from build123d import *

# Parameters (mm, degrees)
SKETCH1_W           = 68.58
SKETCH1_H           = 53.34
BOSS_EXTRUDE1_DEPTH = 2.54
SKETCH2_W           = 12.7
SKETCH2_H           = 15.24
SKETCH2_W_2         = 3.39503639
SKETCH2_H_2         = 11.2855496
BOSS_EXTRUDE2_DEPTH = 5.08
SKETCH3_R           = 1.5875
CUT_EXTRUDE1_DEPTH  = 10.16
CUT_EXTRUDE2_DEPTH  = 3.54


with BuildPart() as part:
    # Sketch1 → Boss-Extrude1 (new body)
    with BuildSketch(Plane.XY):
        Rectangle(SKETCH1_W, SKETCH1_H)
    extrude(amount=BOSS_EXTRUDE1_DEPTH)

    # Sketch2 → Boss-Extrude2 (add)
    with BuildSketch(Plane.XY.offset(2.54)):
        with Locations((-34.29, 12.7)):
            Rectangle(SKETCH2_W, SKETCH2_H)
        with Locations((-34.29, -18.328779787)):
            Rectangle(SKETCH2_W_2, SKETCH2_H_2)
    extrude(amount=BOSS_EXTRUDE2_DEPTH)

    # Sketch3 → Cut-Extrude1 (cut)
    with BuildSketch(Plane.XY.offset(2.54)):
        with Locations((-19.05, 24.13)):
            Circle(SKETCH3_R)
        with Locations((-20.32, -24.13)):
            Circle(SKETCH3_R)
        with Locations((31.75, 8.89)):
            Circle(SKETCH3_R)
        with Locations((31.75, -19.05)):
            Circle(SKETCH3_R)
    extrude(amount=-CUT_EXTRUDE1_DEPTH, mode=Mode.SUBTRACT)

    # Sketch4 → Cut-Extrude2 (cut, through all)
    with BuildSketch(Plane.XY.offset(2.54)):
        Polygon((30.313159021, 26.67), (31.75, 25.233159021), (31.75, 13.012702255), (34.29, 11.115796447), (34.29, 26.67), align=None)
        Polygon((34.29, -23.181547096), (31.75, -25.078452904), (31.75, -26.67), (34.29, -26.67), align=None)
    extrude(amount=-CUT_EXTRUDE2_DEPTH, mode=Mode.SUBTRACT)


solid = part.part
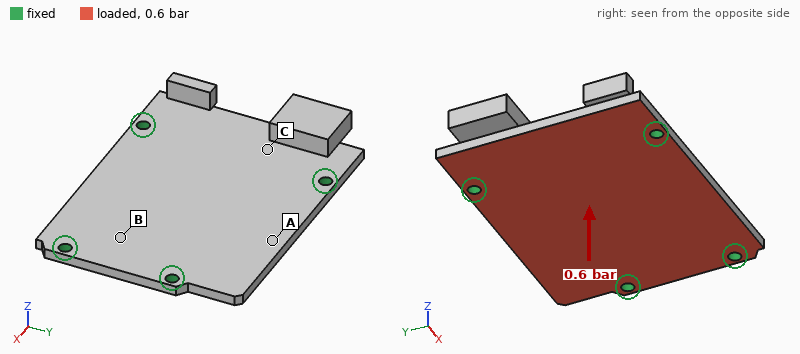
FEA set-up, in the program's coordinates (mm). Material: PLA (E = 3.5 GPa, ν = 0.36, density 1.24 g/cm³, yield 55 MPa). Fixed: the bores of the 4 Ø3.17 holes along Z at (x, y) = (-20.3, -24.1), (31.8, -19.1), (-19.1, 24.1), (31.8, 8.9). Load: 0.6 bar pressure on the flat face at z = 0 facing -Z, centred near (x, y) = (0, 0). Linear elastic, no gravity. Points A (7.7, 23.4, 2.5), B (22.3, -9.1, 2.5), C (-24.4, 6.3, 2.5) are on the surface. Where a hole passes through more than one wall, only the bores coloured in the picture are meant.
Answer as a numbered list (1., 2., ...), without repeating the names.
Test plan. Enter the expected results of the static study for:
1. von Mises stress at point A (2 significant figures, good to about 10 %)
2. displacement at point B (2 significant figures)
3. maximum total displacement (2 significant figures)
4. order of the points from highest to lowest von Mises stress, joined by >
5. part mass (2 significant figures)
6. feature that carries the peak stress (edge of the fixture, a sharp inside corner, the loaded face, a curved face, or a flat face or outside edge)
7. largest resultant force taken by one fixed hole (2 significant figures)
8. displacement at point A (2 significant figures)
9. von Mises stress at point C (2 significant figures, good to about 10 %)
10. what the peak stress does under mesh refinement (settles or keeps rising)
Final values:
1. 8.2 MPa
2. 0.15 mm
3. 0.38 mm
4. A > C > B
5. 13 g
6. edge of the fixture
7. 65 N
8. 0.36 mm
9. 5.1 MPa
10. keeps rising
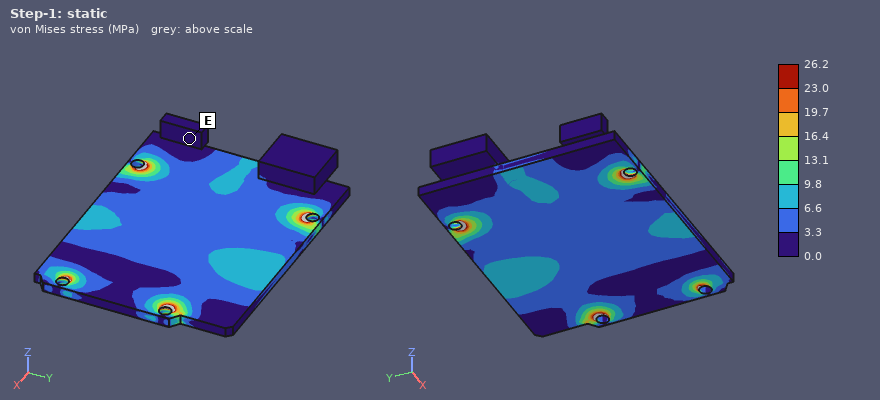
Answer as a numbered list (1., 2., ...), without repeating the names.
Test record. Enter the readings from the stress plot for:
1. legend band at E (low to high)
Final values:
1. 0.0 to 3.3 MPa
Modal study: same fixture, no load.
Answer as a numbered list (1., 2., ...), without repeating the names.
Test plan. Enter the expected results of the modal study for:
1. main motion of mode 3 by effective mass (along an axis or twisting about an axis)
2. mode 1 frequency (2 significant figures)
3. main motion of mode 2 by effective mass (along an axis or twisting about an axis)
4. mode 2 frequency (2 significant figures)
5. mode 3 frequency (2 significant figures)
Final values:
1. twisting about X
2. 1000 Hz
3. along Z
4. 1300 Hz
5. 1600 Hz
